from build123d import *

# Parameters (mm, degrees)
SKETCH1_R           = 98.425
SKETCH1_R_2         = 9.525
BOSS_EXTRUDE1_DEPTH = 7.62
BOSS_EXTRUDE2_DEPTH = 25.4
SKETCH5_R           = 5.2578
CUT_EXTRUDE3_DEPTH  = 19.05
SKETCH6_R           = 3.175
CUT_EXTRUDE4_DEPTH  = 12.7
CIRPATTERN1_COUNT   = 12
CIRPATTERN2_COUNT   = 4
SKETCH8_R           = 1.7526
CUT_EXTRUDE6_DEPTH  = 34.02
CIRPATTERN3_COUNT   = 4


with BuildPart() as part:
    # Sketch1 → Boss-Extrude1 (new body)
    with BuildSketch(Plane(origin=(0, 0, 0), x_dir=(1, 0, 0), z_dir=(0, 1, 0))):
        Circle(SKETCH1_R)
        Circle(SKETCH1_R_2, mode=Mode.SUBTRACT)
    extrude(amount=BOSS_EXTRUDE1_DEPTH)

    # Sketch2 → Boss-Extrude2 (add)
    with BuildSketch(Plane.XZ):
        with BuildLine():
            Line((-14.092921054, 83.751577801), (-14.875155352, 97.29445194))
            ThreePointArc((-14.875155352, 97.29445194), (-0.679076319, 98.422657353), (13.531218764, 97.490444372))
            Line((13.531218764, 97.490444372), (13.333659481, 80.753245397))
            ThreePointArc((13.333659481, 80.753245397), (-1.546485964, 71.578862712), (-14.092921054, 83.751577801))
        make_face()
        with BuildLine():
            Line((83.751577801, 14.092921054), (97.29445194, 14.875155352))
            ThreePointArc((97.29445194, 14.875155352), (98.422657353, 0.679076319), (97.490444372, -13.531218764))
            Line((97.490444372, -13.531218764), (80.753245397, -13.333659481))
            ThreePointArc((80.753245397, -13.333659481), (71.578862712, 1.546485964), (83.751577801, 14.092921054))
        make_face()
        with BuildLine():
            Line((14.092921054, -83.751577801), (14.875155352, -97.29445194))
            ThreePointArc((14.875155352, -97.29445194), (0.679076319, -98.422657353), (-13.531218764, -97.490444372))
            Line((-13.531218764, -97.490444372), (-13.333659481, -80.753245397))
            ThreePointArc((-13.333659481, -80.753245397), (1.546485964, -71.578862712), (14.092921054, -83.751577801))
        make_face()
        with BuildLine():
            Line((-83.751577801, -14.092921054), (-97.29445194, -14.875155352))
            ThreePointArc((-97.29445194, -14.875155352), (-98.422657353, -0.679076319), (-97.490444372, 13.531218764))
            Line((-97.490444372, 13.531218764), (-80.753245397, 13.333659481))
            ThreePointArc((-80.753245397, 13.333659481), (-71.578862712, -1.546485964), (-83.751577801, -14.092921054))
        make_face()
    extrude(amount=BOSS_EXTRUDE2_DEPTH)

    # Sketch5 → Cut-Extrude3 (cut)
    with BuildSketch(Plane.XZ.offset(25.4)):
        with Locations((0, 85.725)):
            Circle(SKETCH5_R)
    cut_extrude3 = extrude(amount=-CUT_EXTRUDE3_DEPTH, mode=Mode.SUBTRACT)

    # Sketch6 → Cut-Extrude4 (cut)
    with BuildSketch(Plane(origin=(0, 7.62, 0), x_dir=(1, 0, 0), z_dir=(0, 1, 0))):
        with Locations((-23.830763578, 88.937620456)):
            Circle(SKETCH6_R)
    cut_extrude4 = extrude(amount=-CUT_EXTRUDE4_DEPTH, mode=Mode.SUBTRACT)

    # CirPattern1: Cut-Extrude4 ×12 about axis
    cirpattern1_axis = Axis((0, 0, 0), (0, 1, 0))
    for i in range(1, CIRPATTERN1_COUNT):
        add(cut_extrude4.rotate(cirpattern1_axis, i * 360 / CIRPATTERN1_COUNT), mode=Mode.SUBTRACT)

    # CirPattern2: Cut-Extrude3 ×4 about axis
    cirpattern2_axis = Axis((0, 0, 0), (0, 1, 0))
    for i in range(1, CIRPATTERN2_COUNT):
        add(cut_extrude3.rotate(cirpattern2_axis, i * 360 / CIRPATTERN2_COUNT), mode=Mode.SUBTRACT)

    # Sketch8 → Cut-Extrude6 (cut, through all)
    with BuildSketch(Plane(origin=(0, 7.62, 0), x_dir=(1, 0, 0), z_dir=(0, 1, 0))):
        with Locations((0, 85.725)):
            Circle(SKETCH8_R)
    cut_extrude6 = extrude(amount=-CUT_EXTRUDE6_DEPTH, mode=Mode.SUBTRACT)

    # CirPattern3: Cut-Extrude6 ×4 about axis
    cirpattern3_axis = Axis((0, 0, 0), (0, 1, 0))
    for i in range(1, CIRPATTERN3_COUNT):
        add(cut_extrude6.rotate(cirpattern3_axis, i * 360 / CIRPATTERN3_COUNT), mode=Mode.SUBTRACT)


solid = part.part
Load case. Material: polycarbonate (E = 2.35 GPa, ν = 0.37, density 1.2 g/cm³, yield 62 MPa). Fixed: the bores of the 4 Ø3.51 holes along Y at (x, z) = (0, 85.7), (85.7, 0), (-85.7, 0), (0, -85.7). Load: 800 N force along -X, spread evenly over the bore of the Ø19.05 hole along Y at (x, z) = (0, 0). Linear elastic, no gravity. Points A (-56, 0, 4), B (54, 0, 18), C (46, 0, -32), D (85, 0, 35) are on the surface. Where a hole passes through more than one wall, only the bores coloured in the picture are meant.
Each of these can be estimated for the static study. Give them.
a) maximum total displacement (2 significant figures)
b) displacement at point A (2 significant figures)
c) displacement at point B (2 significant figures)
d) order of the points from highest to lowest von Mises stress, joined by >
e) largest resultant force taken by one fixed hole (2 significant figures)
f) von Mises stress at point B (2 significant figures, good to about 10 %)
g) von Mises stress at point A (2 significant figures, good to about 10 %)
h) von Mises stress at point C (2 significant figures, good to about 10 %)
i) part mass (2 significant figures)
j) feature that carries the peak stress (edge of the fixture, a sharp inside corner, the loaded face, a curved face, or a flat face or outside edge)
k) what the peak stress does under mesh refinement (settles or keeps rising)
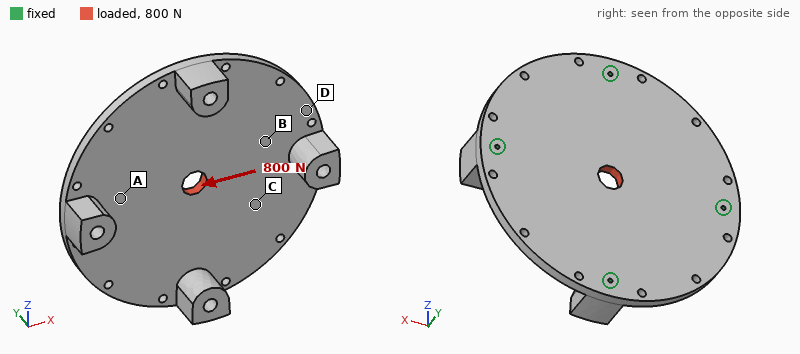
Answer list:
39 µm
17 µm
18 µm
A > B > C > D
260 N
0.73 MPa
1.1 MPa
0.43 MPa
340 g
edge of the fixture
keeps rising
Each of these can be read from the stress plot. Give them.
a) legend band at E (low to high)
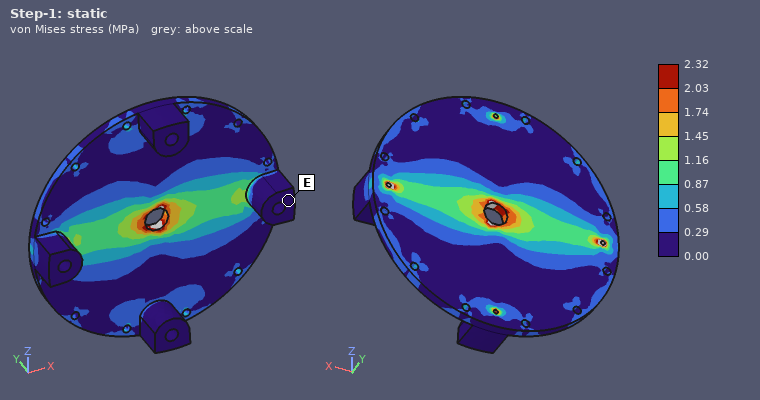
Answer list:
0.00 to 0.29 MPa
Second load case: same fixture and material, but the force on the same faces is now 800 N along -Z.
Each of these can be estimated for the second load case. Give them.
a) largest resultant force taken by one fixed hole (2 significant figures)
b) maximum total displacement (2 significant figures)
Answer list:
260 N
39 µm
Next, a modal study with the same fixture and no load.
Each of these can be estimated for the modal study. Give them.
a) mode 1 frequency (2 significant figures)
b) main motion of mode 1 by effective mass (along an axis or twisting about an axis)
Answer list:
590 Hz
along Y
